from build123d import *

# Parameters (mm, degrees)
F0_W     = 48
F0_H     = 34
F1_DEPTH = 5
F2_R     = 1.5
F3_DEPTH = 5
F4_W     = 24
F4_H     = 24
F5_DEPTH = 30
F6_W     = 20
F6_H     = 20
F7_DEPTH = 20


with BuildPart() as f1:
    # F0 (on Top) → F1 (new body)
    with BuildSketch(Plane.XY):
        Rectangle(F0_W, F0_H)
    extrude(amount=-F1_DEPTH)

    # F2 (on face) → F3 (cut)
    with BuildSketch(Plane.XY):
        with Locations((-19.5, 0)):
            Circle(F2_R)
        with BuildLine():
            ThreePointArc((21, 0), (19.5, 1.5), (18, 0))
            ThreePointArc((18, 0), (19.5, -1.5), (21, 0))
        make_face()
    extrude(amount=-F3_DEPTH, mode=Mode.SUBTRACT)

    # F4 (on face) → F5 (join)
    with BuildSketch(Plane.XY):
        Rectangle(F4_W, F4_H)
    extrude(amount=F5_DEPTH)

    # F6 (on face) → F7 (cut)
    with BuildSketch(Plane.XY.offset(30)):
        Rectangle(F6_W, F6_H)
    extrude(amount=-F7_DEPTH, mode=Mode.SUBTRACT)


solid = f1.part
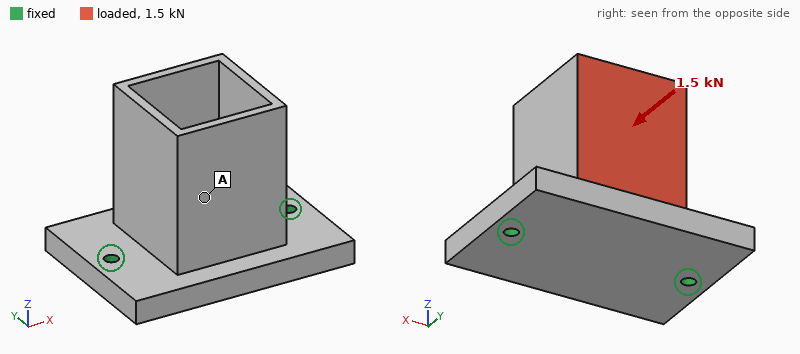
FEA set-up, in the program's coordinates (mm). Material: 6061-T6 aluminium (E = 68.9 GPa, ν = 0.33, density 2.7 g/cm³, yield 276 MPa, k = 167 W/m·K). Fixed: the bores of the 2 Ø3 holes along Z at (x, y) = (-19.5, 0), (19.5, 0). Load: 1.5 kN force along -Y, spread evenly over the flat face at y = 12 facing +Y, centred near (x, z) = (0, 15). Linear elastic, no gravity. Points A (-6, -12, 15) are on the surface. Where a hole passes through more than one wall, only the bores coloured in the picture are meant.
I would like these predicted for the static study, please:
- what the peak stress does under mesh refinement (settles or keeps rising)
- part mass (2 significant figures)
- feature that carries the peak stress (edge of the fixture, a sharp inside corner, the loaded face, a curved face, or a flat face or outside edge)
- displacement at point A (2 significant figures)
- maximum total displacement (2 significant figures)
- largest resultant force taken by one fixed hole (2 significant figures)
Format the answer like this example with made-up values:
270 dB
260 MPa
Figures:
keeps rising
47 g
edge of the fixture
0.12 mm
0.25 mm
750 N
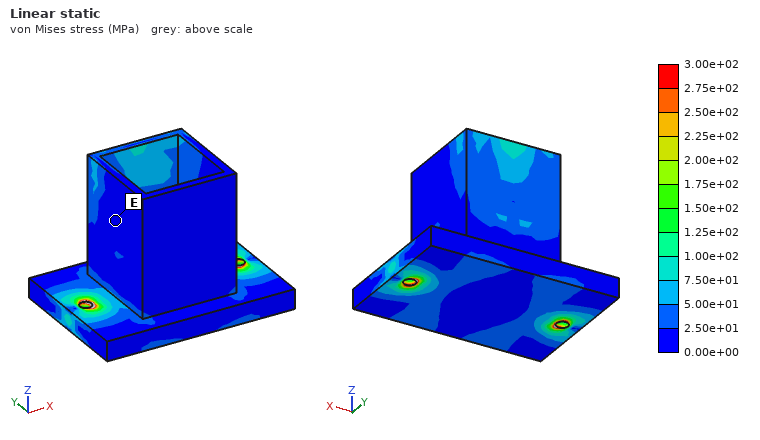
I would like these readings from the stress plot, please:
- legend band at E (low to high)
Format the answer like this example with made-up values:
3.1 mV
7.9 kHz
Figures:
0.00e+00 to 2.50e+01 MPa
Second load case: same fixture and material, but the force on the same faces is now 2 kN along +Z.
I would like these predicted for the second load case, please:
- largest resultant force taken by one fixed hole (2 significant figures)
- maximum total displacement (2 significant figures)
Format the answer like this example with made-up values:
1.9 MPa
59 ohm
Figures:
1.1 kN
0.19 mm
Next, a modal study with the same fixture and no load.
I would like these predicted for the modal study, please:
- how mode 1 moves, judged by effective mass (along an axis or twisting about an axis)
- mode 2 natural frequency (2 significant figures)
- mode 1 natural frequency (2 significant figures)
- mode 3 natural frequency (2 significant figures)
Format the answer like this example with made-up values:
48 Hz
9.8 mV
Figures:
along Y
9400 Hz
3600 Hz
9600 Hz
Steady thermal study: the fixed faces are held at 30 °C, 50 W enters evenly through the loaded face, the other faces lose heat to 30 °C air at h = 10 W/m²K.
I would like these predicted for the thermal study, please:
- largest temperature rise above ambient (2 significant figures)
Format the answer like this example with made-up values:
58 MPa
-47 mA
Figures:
49 K
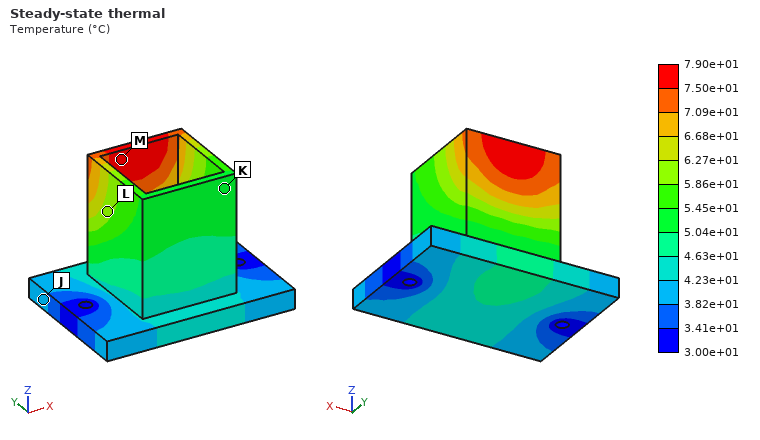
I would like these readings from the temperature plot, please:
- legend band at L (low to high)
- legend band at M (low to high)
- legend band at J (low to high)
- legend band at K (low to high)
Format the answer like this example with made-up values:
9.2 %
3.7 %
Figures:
5.86e+01 to 6.27e+01 °C
7.50e+01 to 7.90e+01 °C
3.82e+01 to 4.23e+01 °C
5.04e+01 to 5.45e+01 °C
